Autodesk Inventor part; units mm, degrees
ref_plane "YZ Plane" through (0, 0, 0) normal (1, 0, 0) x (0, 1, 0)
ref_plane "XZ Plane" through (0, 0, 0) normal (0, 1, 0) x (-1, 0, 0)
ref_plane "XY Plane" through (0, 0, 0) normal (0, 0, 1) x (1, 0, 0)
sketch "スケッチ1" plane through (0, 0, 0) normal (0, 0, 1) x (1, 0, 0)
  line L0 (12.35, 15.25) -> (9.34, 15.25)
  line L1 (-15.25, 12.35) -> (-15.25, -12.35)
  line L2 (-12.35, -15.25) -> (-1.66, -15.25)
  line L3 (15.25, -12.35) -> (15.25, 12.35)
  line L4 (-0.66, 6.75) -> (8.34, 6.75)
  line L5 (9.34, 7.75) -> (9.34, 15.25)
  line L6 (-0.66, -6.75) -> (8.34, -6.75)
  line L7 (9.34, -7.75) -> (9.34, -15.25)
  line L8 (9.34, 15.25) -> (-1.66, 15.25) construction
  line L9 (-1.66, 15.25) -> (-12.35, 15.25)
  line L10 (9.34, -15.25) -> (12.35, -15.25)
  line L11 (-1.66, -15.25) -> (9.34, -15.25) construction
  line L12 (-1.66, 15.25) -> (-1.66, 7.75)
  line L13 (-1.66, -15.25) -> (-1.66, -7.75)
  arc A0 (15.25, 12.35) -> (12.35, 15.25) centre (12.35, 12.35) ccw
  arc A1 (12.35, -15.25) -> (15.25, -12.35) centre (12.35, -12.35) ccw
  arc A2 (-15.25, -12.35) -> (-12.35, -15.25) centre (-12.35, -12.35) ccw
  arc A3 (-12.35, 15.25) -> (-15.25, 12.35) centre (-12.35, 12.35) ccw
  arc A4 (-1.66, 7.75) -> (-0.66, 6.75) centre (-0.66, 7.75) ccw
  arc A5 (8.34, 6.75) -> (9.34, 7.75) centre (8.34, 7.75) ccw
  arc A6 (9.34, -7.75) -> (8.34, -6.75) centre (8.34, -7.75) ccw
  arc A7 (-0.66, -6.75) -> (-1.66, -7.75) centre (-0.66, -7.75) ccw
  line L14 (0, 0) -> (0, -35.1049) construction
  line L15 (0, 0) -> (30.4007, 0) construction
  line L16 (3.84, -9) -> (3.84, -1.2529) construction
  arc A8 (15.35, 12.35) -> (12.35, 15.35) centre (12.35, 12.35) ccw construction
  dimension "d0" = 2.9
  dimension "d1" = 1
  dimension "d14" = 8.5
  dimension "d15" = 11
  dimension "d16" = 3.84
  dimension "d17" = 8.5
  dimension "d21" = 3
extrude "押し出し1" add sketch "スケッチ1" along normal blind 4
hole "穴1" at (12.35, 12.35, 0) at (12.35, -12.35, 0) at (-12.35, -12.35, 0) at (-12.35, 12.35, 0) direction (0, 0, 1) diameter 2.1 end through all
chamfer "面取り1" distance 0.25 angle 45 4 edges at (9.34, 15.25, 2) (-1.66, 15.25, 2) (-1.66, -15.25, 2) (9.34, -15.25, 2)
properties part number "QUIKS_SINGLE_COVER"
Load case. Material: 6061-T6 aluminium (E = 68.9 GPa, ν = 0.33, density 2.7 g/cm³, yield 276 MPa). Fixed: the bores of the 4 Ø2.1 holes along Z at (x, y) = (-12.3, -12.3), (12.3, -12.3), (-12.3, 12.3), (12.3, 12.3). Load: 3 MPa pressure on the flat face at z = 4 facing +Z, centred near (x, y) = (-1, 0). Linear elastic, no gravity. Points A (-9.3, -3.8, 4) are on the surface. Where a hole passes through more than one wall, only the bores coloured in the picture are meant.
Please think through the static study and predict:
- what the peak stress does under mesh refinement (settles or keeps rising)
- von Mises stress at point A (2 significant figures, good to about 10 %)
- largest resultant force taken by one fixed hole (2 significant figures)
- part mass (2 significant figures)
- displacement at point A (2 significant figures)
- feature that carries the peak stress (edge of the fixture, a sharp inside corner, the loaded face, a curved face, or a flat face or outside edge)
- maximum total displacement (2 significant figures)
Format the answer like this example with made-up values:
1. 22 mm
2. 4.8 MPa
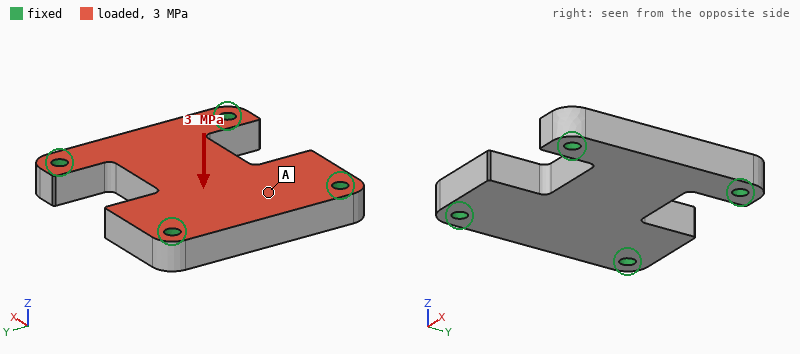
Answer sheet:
1. keeps rising
2. 25 MPa
3. 640 N
4. 7.8 g
5. 18 µm
6. edge of the fixture
7. 30 µm
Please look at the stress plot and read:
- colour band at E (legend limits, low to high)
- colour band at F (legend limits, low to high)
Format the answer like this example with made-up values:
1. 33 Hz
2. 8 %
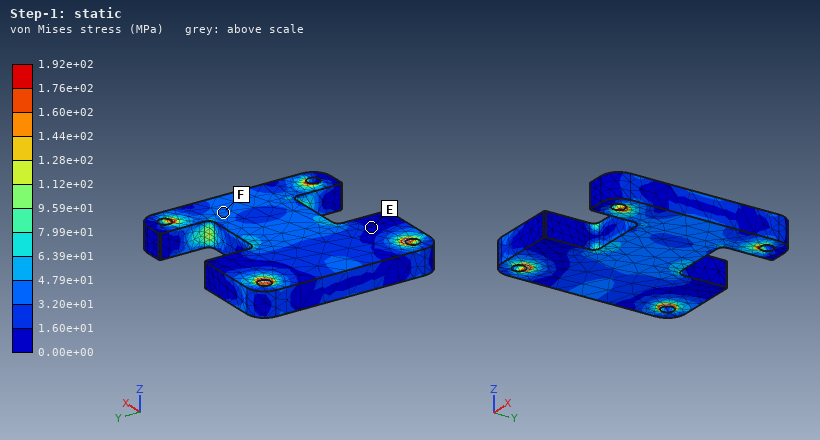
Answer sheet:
1. 0.00e+00 to 1.60e+01 MPa
2. 3.20e+01 to 4.79e+01 MPa
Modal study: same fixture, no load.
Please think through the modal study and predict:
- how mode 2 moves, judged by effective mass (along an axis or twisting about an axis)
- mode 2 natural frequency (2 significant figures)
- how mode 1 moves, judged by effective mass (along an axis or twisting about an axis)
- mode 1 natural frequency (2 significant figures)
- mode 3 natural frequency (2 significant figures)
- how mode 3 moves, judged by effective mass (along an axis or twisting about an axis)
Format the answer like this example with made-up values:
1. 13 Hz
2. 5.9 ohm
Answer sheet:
1. twisting about Y
2. 30 kHz
3. along Z
4. 18 kHz
5. 32 kHz
6. twisting about X
